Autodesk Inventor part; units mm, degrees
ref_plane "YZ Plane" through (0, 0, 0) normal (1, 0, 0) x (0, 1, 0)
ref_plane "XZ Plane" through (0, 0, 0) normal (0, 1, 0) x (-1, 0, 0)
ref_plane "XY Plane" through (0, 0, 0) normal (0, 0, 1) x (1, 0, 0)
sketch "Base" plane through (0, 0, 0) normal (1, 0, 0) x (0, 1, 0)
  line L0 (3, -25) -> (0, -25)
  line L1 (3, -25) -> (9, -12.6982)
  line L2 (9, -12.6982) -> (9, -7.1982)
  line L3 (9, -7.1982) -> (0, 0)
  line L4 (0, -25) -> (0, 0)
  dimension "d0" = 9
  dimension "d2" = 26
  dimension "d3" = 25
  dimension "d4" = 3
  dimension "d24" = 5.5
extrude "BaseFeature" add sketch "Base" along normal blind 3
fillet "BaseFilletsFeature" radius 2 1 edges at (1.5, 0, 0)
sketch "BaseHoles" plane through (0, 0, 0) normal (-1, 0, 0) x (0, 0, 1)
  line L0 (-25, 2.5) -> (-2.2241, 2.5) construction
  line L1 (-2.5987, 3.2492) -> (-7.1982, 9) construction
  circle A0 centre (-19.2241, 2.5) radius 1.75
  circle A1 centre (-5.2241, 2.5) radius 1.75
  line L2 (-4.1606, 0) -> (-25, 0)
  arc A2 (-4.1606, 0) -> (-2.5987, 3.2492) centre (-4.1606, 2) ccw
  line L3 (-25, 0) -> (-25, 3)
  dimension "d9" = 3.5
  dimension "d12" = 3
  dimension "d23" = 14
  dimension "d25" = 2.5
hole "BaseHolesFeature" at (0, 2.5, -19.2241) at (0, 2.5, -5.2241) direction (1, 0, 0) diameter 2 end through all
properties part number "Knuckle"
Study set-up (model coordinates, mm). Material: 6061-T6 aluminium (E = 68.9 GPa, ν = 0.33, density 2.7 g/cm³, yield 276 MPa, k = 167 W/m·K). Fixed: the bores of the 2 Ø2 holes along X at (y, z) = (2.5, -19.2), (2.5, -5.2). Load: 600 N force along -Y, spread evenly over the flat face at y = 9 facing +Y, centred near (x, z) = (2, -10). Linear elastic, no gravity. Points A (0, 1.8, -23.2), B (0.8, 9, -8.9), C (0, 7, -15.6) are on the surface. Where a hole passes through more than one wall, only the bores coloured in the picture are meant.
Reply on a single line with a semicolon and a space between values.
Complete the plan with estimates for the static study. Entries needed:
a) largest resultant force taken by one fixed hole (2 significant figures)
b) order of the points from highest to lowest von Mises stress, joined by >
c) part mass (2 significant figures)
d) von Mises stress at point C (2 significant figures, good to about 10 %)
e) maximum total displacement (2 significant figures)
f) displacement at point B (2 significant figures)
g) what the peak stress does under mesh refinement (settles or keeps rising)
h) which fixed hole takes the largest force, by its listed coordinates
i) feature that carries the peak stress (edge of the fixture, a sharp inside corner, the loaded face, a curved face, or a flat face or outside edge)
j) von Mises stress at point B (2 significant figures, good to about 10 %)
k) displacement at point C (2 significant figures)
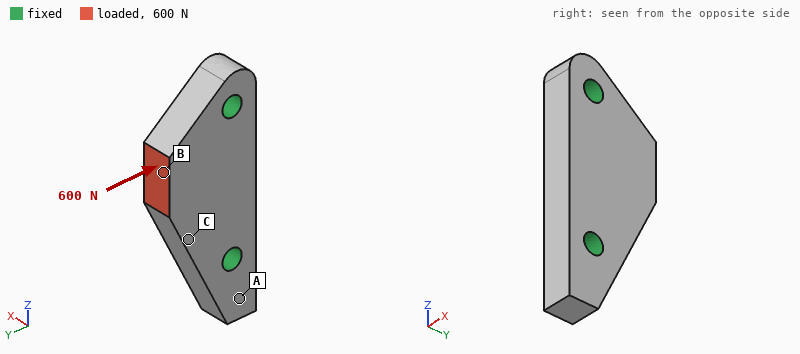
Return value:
420 N; B > C > A; 1.2 g; 19 MPa; 4.9 µm; 4.4 µm; keeps rising; (2.5, -5.2); edge of the fixture; 35 MPa; 2.0 µm
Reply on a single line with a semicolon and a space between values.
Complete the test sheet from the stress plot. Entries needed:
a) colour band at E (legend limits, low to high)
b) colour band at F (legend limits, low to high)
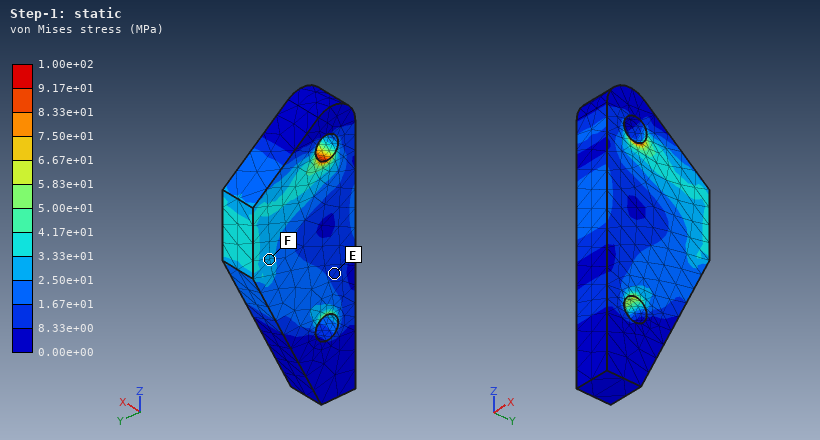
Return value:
8.33e+00 to 1.67e+01 MPa; 2.50e+01 to 3.33e+01 MPa
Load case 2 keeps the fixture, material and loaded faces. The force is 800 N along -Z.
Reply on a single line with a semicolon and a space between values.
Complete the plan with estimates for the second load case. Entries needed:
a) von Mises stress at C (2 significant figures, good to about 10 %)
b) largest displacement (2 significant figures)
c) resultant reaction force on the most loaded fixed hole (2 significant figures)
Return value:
54 MPa; 8.8 µm; 540 N
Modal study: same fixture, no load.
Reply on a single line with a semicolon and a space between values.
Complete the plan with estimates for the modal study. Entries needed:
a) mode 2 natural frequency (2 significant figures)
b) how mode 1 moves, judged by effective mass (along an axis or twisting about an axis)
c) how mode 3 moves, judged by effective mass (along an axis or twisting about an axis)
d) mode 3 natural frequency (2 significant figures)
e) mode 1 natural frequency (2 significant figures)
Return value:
74 kHz; along X; along X; 81 kHz; 43 kHz
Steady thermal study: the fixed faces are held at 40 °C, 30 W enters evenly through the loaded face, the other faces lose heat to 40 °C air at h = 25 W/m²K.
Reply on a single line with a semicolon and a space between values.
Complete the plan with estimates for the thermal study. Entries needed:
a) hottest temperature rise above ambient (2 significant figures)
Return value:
53 K
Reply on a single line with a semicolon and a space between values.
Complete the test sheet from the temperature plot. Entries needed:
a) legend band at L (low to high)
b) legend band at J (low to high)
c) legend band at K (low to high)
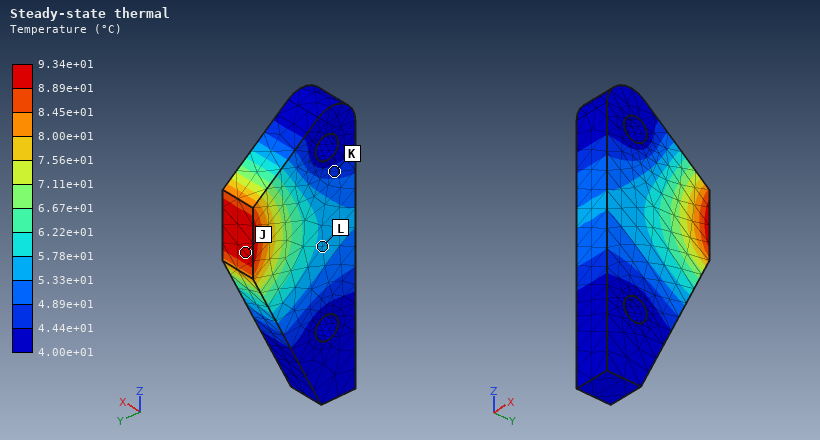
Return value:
5.33e+01 to 5.78e+01 °C; 8.89e+01 to 9.34e+01 °C; 4.44e+01 to 4.89e+01 °C
